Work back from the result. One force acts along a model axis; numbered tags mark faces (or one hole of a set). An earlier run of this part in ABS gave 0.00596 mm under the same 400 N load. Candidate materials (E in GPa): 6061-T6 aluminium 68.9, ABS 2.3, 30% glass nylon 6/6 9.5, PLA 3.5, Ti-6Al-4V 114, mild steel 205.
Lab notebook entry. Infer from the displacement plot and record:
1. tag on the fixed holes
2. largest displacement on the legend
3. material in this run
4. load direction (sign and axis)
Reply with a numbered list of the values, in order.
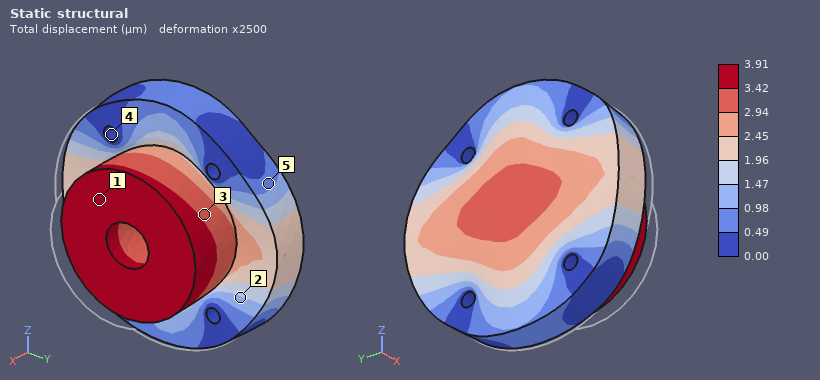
1. 4
2. 3.91 µm
3. PLA
4. -X
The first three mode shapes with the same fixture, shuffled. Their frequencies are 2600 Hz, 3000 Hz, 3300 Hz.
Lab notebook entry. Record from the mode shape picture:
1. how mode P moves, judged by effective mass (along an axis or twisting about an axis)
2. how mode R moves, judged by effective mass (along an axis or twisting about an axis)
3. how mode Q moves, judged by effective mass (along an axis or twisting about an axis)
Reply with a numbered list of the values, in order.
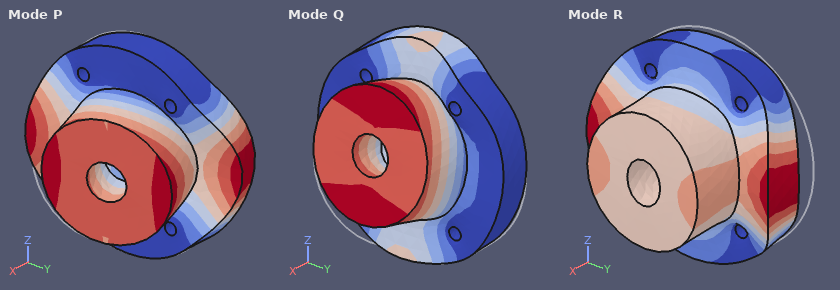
1. along Y
2. along X
3. along Z
